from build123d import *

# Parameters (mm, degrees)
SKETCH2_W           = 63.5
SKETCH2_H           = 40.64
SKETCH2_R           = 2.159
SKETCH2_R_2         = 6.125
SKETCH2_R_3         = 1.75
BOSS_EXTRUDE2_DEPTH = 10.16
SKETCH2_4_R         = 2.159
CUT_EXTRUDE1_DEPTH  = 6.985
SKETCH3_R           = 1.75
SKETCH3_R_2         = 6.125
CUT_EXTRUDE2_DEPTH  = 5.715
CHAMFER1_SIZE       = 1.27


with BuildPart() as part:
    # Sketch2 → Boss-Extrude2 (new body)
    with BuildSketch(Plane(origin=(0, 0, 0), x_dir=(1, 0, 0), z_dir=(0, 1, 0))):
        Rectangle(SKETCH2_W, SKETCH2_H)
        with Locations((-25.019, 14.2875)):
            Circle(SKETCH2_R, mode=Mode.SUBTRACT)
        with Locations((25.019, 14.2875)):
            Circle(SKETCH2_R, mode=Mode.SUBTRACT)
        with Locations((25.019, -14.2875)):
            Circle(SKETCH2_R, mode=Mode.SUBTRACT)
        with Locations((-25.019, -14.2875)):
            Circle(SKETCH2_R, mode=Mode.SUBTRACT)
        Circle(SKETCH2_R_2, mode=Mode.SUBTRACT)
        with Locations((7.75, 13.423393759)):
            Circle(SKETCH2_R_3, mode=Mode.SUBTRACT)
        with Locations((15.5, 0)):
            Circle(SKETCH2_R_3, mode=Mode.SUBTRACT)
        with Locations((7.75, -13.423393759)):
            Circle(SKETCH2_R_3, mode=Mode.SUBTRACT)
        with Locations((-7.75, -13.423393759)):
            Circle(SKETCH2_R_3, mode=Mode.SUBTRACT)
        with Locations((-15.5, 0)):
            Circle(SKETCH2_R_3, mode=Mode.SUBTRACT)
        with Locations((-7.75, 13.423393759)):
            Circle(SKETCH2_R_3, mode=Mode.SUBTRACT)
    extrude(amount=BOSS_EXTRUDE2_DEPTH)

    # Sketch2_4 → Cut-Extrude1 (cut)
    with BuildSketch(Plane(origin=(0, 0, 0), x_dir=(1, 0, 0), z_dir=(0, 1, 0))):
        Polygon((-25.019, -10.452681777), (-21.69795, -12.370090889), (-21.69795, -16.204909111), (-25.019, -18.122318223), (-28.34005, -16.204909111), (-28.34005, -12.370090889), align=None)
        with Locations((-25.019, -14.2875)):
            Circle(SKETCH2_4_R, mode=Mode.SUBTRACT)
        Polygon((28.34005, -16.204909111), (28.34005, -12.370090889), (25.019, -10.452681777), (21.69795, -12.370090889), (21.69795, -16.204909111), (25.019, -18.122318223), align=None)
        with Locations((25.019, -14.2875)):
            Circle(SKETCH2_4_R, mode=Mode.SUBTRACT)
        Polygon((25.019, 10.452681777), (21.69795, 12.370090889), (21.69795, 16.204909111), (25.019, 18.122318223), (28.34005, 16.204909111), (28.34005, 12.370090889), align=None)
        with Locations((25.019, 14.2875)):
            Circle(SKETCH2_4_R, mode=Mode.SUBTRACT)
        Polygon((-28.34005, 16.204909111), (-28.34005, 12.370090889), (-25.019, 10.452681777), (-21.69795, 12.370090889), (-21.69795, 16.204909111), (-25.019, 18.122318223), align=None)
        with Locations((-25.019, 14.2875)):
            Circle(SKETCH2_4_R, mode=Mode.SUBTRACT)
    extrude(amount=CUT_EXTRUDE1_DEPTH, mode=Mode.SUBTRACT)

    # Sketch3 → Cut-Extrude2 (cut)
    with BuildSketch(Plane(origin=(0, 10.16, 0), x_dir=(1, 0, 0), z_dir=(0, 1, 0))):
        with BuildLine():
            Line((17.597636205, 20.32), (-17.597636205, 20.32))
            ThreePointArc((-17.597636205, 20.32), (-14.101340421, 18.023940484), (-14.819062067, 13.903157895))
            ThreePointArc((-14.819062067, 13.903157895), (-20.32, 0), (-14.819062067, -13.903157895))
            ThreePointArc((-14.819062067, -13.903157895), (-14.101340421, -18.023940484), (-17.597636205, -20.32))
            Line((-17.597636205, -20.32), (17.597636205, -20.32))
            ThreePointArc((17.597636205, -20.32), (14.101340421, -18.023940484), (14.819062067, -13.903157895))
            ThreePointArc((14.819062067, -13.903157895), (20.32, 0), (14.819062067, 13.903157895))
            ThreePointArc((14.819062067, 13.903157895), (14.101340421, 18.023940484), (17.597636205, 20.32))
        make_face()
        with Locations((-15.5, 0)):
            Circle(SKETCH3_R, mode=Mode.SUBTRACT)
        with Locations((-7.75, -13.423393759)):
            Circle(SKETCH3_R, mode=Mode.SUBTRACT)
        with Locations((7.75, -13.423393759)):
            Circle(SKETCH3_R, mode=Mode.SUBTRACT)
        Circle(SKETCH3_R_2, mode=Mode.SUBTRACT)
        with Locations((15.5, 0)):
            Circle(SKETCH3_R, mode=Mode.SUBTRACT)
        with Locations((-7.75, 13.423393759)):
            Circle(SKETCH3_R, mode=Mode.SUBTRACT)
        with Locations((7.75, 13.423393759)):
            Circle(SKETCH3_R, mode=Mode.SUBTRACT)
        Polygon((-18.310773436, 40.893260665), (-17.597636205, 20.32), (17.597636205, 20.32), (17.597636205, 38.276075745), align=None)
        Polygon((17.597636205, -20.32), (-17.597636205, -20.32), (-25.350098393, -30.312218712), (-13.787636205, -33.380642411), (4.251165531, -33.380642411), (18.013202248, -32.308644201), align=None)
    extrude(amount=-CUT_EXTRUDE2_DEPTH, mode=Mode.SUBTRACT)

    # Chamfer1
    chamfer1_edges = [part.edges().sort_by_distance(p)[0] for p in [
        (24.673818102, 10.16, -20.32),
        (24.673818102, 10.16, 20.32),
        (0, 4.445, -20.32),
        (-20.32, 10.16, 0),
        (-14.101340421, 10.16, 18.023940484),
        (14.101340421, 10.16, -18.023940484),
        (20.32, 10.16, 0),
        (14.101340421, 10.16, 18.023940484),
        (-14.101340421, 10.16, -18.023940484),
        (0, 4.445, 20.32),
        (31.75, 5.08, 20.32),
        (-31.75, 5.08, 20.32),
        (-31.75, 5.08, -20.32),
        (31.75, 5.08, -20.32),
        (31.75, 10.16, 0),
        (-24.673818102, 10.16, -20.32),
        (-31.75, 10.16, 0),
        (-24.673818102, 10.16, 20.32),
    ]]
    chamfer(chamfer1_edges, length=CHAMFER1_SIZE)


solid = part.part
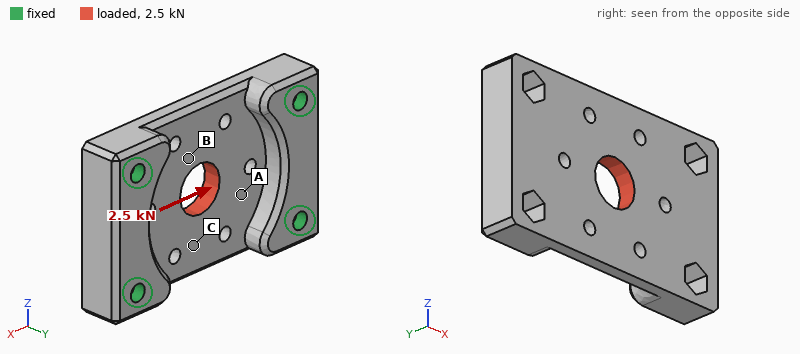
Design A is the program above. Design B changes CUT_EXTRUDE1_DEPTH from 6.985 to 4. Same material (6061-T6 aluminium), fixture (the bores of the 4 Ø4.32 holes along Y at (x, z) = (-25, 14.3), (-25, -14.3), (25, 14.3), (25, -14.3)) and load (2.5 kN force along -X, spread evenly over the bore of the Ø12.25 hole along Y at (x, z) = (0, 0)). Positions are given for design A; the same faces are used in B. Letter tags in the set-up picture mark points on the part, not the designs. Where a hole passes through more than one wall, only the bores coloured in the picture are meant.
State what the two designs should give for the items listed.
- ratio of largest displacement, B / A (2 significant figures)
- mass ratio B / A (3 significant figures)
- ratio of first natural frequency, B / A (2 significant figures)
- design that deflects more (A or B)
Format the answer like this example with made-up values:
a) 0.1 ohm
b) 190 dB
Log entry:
a) 0.57
b) 1.02
c) 1.1
d) A
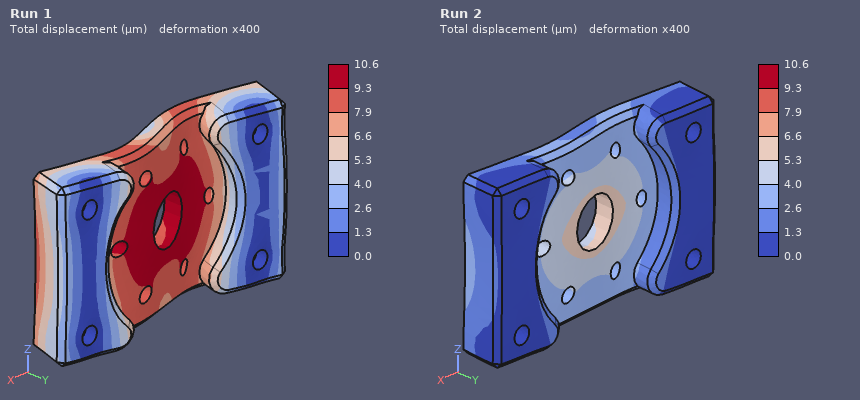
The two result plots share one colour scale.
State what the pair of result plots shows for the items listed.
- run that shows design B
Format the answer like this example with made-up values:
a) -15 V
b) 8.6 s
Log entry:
a) Run 2
